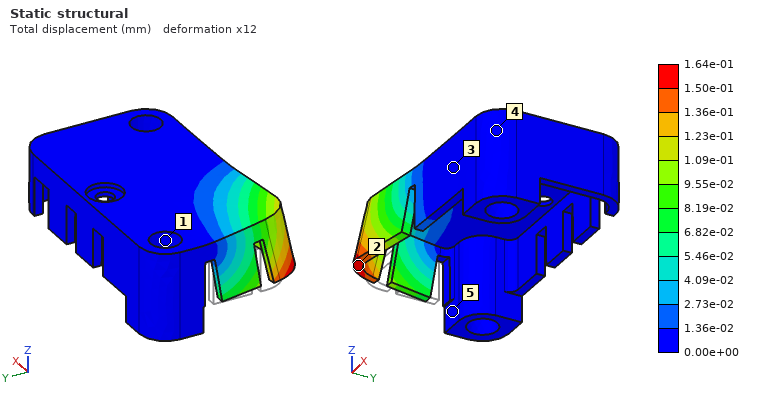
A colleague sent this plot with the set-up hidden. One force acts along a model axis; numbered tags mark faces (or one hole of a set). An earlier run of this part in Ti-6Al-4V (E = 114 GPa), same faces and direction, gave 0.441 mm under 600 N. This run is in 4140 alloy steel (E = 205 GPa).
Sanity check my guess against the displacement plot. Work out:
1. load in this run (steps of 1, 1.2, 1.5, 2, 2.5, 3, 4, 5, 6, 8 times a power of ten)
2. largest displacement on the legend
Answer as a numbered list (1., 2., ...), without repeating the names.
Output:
1. 400 N
2. 1.64e-01 mm
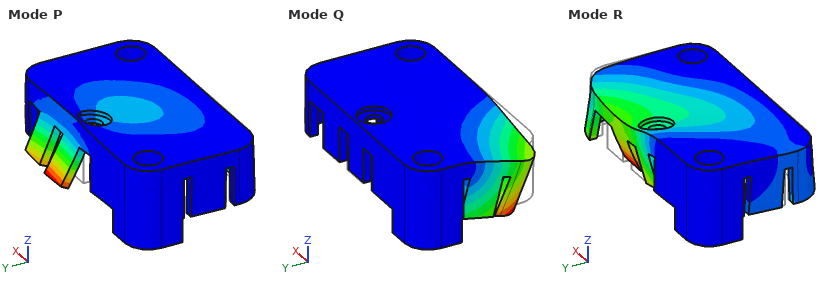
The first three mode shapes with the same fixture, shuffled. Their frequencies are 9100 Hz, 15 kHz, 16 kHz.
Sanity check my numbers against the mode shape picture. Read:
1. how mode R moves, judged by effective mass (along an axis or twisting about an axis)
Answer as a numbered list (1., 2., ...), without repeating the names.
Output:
1. along Z
